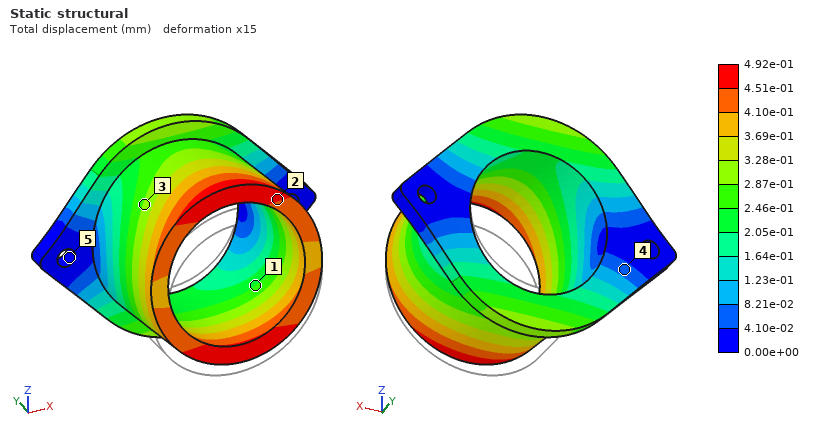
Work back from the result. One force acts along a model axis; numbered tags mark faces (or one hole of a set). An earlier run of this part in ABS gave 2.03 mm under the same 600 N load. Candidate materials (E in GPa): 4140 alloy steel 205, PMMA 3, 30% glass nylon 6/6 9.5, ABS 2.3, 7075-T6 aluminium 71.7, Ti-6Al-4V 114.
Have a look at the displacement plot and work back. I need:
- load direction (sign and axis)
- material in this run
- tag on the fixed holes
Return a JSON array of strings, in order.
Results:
["+Z", "30% glass nylon 6/6", "5"]
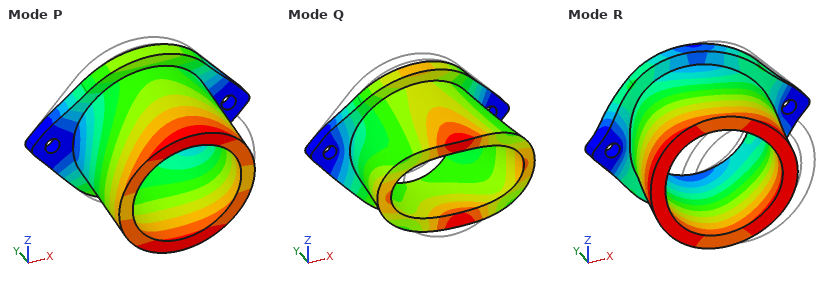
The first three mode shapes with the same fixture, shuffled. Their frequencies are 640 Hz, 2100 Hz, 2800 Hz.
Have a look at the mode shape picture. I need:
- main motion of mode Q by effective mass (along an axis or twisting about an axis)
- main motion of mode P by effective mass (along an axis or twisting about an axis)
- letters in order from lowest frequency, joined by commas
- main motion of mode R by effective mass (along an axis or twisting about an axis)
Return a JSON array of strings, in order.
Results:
["along Y", "along Z", "P, Q, R", "along X"]
